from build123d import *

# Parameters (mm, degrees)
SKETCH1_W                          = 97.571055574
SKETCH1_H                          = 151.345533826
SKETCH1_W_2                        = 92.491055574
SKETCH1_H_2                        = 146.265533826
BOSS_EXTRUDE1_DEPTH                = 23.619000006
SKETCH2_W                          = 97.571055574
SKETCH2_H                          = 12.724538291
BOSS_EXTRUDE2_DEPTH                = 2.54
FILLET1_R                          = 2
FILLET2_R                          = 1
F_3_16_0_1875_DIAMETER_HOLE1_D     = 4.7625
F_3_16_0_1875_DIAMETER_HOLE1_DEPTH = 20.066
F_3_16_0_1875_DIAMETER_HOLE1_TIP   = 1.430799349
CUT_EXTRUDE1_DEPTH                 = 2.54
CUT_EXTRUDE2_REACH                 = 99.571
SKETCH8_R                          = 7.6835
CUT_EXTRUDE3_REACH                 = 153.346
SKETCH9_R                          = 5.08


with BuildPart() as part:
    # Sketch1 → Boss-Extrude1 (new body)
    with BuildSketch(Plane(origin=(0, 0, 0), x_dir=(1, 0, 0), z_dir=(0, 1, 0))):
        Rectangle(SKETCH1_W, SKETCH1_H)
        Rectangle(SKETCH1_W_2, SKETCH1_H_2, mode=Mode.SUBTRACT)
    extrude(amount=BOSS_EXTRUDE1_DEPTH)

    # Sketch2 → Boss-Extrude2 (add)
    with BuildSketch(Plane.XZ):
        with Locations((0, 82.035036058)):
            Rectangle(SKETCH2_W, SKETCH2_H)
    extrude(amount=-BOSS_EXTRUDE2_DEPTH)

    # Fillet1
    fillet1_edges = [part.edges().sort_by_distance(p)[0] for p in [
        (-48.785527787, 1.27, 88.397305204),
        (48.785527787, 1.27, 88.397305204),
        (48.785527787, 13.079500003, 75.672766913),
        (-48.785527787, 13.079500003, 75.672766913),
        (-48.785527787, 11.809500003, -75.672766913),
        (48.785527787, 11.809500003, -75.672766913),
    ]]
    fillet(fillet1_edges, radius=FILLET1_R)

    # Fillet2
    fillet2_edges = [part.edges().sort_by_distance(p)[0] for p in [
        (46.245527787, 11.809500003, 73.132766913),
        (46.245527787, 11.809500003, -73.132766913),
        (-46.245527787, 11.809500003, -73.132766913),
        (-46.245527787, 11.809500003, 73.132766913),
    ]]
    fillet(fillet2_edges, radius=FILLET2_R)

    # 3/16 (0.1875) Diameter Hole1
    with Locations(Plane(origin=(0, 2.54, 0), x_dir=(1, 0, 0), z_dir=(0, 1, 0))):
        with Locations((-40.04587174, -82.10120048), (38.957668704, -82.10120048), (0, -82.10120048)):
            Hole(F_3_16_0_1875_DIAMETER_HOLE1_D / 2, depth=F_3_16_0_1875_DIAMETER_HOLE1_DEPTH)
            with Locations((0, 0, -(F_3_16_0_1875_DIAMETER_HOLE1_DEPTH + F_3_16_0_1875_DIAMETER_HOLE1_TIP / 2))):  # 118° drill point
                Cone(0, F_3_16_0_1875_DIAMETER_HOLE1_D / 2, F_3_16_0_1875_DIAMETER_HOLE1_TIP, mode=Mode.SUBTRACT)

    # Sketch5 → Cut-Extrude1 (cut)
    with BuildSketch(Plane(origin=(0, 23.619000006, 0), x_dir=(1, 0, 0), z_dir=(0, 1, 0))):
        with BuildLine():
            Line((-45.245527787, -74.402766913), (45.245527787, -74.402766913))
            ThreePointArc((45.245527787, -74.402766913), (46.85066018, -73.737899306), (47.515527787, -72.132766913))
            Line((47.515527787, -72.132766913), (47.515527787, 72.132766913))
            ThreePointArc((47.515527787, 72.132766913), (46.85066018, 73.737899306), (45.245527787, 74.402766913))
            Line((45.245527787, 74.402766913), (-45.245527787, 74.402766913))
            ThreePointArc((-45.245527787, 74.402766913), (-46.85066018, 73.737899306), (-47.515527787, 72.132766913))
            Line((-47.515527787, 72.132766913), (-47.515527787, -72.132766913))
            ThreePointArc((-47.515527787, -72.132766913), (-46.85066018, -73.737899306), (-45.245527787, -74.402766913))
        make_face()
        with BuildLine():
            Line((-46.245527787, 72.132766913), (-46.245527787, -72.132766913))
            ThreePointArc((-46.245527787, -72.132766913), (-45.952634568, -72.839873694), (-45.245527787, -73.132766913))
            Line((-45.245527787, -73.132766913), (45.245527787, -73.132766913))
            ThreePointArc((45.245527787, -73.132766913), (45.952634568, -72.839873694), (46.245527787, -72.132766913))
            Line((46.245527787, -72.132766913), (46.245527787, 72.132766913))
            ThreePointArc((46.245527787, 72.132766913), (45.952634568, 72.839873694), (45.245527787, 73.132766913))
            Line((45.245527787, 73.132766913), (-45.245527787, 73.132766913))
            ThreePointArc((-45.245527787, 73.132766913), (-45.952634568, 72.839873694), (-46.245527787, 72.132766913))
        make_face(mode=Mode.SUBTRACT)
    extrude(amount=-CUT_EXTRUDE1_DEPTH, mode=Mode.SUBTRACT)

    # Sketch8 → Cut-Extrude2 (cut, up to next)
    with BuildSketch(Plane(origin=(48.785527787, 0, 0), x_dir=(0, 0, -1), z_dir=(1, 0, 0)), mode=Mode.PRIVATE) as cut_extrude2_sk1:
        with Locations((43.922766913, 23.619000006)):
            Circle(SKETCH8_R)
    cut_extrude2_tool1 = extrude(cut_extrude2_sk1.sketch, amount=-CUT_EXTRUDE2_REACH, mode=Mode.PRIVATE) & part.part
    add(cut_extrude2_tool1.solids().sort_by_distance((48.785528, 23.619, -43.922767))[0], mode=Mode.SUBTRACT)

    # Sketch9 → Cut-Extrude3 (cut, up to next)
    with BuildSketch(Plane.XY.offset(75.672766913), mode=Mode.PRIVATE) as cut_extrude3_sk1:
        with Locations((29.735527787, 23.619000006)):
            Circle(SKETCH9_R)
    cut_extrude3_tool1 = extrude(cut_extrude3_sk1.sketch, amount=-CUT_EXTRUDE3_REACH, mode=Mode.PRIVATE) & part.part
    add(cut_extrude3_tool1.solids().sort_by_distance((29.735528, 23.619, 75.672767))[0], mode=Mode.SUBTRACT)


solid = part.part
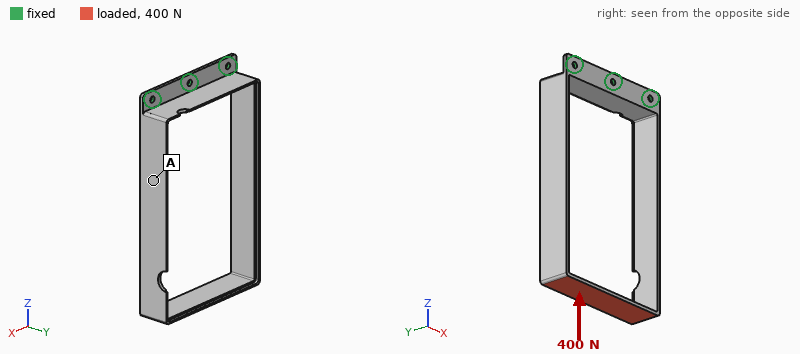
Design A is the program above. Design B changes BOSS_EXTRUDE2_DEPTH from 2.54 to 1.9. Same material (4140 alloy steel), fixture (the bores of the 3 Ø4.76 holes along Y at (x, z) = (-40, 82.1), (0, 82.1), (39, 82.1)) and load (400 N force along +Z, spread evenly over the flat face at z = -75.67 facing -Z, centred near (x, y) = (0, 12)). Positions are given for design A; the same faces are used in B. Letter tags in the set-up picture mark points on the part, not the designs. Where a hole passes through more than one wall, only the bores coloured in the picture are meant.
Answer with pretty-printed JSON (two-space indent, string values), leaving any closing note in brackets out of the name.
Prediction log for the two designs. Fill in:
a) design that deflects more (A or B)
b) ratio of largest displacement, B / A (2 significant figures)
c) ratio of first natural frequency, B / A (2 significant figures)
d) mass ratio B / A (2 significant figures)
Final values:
{
  "design that deflects more": "B",
  "ratio of largest displacement, B / A": "1.4",
  "ratio of first natural frequency, B / A": "0.99",
  "mass ratio B / A": "0.97"
}
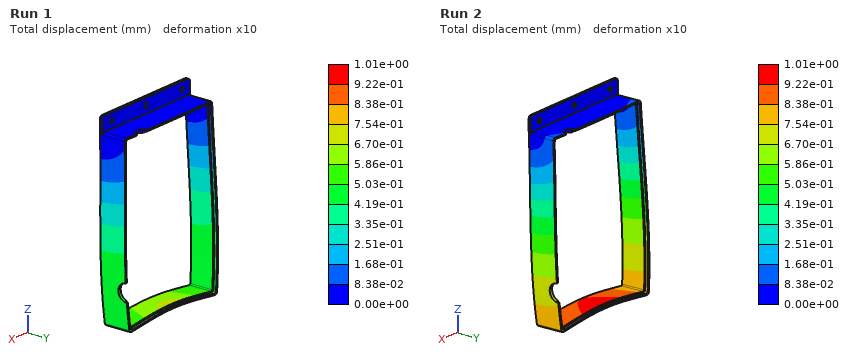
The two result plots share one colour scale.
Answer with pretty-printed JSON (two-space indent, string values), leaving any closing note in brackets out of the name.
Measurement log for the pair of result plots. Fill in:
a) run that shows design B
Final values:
{
  "run that shows design B": "Run 2"
}
